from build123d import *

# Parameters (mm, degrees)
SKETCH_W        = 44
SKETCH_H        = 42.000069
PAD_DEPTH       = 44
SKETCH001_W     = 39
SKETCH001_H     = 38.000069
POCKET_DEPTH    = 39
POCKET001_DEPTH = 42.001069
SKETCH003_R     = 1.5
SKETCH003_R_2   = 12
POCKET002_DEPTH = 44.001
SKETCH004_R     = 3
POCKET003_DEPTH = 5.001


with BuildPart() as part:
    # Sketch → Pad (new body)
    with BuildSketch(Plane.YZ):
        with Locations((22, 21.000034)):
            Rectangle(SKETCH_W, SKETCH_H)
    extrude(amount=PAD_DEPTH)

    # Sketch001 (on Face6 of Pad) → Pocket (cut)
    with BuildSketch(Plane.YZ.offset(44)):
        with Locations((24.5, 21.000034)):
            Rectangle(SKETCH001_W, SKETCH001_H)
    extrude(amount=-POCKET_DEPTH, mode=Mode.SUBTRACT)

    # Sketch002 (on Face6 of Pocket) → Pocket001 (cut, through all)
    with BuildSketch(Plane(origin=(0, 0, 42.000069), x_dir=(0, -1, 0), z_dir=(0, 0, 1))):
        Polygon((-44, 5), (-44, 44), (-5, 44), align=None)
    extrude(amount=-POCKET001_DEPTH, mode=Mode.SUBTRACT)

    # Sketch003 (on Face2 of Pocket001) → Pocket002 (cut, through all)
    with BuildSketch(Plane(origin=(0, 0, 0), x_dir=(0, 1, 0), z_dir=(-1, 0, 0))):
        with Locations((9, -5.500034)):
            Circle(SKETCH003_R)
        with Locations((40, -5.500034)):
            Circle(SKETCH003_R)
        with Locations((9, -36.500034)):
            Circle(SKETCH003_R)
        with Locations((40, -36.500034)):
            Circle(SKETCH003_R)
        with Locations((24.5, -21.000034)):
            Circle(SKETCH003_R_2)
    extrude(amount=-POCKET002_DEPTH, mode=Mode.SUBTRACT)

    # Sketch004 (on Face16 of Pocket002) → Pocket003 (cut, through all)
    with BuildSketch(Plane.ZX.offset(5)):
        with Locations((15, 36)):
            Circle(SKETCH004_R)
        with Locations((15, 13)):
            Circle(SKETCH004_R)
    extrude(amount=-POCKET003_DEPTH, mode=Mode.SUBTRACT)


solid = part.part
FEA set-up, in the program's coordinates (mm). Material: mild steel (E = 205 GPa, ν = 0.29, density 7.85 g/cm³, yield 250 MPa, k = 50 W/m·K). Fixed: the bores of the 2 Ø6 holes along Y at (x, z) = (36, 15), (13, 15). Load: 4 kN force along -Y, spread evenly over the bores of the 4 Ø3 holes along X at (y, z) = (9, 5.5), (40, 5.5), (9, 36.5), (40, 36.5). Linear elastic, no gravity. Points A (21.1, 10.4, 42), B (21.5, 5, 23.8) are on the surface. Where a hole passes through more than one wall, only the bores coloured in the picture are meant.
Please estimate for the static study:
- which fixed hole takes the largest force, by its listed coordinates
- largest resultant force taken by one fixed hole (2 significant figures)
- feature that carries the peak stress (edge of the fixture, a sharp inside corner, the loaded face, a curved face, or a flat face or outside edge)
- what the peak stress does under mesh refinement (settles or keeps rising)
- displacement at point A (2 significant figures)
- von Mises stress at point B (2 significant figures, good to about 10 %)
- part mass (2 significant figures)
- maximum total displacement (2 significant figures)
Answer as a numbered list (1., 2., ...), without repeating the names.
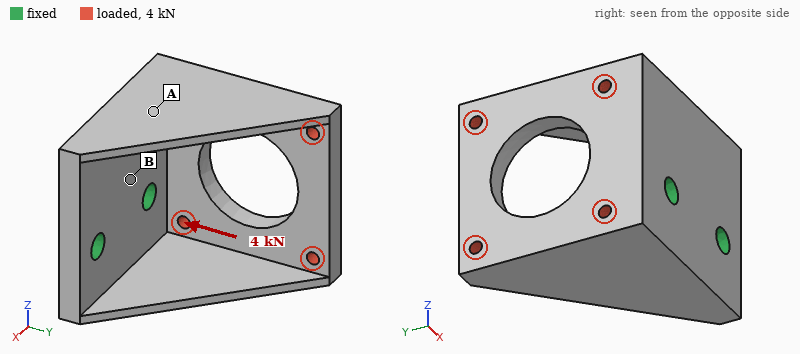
1. (13, 15)
2. 4.7 kN
3. edge of the fixture
4. keeps rising
5. 0.042 mm
6. 75 MPa
7. 140 g
8. 0.12 mm
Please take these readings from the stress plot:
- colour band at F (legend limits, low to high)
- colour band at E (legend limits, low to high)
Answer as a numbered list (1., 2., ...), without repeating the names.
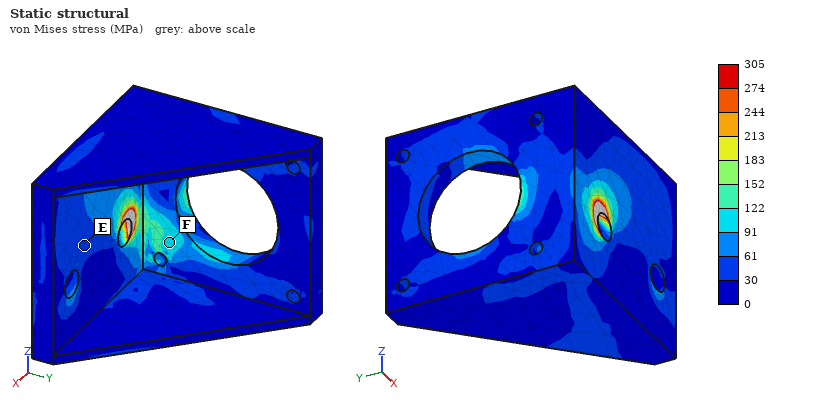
1. 91 to 122 MPa
2. 30 to 61 MPa
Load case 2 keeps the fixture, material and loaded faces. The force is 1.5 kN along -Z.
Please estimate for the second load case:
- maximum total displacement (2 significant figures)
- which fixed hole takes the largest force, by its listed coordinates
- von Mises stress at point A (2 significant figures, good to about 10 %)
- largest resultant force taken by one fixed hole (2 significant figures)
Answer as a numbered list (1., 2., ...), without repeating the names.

1. 0.12 mm
2. (13, 15)
3. 20 MPa
4. 1.9 kN
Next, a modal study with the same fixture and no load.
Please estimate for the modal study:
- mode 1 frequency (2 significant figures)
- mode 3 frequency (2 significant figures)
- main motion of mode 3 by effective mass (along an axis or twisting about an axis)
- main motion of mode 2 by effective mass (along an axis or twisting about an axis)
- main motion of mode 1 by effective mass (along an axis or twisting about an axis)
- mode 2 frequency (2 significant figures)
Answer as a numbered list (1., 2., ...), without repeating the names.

1. 2500 Hz
2. 6100 Hz
3. along Y
4. along X
5. along Z
6. 3800 Hz
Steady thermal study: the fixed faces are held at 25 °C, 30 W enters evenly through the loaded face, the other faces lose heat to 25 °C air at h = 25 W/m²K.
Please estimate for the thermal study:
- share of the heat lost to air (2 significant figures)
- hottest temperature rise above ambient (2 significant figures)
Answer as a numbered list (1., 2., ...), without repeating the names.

1. 27 %
2. 84 K
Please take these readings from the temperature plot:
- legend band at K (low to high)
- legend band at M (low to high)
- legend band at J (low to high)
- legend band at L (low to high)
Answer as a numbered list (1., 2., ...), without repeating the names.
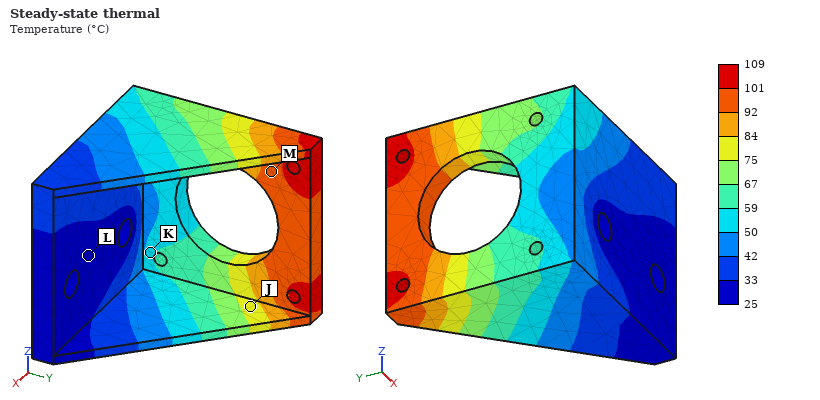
1. 50 to 59 °C
2. 92 to 101 °C
3. 75 to 84 °C
4. 25 to 33 °C
